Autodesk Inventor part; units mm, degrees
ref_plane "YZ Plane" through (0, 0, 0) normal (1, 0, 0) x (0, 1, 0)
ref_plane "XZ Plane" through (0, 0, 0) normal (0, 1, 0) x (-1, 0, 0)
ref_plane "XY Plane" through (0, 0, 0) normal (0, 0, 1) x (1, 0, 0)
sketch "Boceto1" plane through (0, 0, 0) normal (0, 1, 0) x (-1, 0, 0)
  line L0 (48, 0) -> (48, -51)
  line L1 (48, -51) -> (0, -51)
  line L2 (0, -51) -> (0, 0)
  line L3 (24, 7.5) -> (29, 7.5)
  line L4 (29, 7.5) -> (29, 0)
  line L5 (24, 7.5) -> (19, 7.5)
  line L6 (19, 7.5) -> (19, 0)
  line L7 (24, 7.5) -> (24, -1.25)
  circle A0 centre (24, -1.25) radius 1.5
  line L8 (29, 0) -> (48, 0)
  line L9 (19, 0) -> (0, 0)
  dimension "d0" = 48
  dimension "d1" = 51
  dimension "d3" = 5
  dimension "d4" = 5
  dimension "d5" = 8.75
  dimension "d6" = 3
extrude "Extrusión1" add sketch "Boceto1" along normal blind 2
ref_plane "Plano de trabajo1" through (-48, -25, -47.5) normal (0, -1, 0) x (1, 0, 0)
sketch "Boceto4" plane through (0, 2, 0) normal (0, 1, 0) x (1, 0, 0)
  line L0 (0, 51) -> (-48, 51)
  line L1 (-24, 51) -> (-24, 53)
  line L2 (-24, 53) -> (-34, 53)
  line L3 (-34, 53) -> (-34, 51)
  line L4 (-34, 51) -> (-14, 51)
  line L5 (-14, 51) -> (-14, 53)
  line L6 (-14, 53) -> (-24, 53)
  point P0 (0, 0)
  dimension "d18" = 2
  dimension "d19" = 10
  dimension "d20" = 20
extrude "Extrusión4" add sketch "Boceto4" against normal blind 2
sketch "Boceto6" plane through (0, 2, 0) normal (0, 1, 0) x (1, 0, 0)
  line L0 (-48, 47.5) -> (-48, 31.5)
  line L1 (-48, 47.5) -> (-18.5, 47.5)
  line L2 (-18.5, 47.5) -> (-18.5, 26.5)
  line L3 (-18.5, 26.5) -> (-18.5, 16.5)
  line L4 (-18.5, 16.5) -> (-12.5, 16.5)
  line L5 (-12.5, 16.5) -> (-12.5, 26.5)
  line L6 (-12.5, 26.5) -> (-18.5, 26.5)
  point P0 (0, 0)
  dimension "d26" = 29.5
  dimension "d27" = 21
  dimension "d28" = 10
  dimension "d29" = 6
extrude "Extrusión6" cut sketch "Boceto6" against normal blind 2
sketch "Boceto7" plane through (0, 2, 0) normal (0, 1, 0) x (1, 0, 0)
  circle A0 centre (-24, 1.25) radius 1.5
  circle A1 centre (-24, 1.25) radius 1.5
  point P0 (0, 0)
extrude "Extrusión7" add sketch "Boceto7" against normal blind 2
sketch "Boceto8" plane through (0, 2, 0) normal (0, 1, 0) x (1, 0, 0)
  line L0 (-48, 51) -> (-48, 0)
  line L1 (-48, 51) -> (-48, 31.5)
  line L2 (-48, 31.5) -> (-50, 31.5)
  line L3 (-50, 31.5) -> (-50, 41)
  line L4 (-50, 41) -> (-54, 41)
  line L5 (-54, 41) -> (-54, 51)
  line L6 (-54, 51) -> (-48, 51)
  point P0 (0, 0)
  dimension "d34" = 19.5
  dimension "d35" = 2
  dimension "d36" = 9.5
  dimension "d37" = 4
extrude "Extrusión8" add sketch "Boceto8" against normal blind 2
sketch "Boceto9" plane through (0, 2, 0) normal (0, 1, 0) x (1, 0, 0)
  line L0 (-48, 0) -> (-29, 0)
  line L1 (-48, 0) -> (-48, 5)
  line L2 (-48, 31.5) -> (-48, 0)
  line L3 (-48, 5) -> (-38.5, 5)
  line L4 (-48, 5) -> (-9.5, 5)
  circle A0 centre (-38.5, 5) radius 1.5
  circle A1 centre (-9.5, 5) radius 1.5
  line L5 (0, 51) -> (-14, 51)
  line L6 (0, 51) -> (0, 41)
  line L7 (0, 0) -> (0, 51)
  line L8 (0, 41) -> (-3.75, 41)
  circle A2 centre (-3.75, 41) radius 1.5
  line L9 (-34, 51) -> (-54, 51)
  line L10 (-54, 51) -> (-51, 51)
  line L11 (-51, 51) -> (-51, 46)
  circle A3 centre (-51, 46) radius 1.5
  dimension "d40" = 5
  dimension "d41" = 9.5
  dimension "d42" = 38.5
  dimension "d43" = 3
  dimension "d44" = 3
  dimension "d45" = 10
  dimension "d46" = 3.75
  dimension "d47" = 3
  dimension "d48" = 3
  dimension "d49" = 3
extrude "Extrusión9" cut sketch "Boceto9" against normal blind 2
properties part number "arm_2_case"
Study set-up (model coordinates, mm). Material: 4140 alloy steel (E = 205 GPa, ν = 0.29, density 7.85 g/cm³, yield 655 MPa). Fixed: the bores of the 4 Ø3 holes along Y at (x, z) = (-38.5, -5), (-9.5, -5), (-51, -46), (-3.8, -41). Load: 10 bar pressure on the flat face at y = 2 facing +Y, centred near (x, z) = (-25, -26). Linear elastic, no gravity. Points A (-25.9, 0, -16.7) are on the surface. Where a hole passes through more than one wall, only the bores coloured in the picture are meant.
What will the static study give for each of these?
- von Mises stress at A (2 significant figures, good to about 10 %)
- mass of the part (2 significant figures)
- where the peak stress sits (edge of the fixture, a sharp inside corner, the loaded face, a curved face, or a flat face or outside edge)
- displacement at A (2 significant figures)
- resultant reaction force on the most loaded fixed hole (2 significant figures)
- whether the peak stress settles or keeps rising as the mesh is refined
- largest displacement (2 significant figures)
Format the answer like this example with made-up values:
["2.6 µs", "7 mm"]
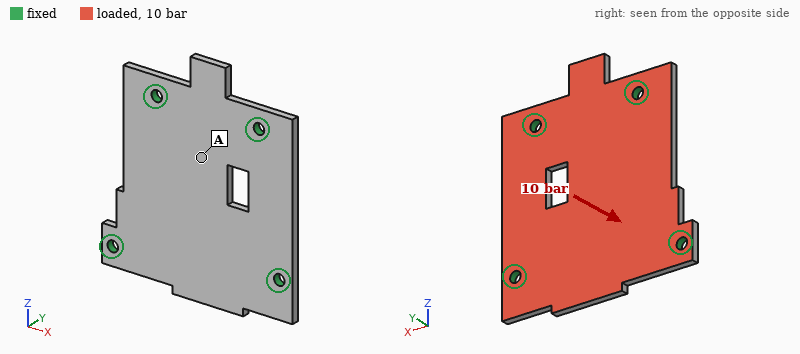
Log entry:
["63 MPa", "40 g", "edge of the fixture", "0.070 mm", "740 N", "keeps rising", "0.12 mm"]
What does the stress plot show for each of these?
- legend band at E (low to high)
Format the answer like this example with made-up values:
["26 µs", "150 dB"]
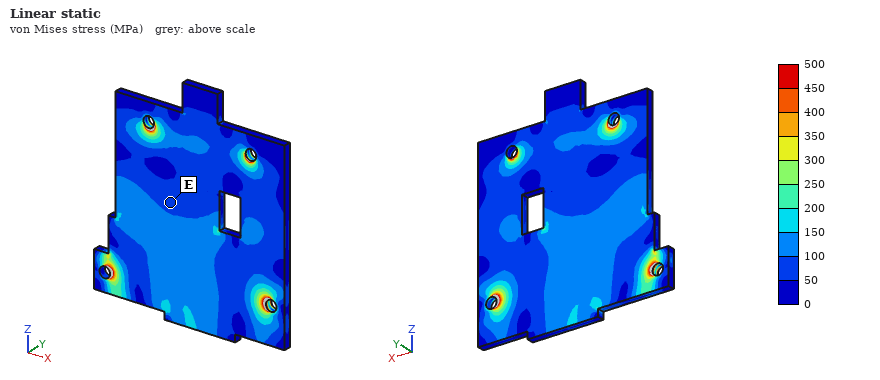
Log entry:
["50 to 100 MPa"]
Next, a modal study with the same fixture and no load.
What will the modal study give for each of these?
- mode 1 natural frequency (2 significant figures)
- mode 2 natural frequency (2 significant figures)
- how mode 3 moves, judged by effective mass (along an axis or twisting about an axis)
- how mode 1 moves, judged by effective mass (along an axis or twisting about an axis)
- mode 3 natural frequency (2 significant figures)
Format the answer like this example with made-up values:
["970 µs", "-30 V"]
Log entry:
["4200 Hz", "5800 Hz", "twisting about Z", "along Y", "7700 Hz"]
